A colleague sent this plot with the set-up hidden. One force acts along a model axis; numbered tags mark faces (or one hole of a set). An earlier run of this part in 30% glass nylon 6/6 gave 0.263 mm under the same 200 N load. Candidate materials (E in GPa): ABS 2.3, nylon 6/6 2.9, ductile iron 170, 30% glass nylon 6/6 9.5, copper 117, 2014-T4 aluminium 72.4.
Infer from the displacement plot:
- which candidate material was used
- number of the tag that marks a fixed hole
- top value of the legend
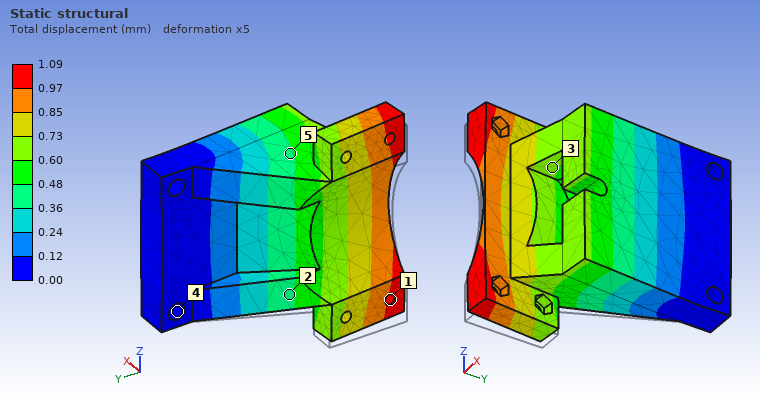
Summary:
ABS
4
1.09 mm
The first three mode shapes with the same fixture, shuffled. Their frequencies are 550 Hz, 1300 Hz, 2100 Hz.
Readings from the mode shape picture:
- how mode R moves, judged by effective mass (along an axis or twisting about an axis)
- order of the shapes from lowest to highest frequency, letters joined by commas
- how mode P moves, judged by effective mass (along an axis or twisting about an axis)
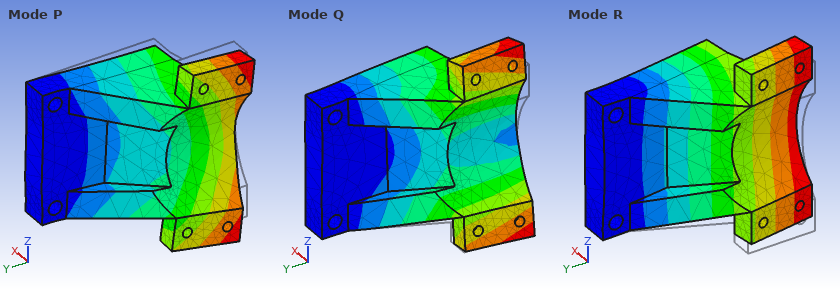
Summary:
along X
R, Q, P
along Z
